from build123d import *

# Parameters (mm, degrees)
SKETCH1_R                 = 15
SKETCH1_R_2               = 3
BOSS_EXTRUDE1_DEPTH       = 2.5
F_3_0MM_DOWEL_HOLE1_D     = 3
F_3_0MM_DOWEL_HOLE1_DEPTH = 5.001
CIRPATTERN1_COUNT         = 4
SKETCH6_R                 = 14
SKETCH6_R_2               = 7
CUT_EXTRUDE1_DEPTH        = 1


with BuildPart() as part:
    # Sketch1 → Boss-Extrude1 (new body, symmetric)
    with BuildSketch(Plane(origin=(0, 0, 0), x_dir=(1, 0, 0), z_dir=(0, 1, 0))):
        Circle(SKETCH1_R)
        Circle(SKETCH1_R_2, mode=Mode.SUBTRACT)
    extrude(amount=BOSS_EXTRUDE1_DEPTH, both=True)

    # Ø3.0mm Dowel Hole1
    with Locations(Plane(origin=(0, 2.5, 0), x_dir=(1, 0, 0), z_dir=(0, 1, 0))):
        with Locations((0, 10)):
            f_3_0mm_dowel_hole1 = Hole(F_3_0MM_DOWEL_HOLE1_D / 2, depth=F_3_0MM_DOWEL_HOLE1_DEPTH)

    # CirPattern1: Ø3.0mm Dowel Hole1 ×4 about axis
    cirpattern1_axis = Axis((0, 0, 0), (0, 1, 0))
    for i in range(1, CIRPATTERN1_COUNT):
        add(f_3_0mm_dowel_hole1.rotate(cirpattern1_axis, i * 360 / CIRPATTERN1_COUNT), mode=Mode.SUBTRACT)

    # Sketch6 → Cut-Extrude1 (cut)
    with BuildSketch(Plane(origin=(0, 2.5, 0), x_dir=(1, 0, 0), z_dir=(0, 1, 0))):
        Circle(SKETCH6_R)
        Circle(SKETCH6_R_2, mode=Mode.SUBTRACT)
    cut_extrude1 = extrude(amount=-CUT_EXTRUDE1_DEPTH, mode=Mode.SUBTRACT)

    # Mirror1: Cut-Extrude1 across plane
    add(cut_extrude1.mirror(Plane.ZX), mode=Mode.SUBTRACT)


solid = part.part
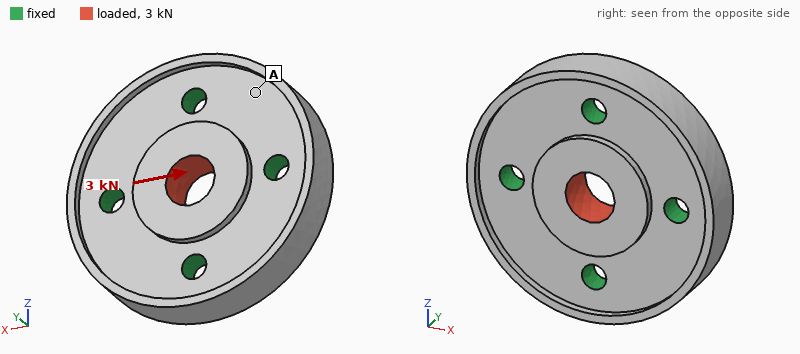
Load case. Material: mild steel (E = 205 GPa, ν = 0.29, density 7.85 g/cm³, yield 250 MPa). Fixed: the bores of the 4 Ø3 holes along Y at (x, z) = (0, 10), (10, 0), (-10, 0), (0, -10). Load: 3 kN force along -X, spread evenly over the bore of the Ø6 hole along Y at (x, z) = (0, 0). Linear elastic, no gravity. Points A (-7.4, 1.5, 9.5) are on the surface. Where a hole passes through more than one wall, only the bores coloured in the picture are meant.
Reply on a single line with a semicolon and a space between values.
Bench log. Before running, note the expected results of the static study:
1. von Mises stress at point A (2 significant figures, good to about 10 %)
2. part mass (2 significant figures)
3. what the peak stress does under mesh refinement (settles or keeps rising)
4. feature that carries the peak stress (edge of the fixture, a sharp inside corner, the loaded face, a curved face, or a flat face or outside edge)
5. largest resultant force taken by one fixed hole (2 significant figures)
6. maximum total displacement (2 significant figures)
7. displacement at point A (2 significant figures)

8.0 MPa; 19 g; keeps rising; edge of the fixture; 980 N; 1.5 µm; 0.44 µm
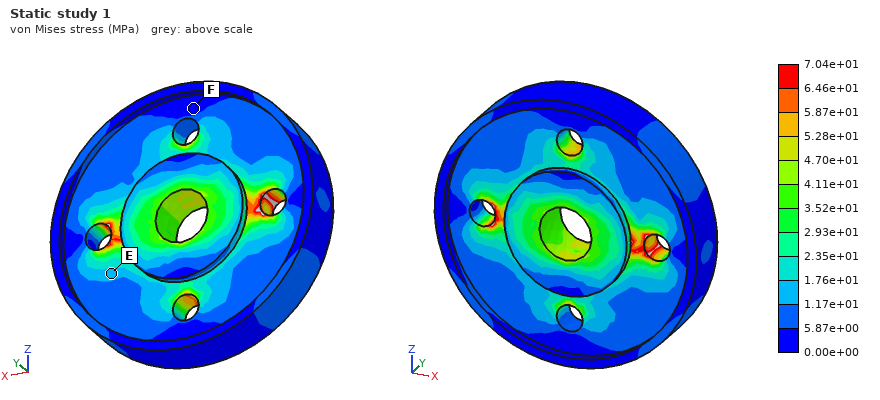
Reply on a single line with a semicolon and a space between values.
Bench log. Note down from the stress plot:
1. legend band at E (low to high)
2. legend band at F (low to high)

1.17e+01 to 1.76e+01 MPa; 0.00e+00 to 5.87e+00 MPa
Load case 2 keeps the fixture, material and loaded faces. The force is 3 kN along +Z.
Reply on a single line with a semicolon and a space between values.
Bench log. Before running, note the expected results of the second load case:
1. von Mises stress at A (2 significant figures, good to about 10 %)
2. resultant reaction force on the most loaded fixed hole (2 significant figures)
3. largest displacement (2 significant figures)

7.5 MPa; 980 N; 1.5 µm
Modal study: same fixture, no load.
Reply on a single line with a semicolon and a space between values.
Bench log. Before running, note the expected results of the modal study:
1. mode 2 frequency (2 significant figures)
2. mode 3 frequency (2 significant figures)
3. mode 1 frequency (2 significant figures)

41 kHz; 41 kHz; 37 kHz
